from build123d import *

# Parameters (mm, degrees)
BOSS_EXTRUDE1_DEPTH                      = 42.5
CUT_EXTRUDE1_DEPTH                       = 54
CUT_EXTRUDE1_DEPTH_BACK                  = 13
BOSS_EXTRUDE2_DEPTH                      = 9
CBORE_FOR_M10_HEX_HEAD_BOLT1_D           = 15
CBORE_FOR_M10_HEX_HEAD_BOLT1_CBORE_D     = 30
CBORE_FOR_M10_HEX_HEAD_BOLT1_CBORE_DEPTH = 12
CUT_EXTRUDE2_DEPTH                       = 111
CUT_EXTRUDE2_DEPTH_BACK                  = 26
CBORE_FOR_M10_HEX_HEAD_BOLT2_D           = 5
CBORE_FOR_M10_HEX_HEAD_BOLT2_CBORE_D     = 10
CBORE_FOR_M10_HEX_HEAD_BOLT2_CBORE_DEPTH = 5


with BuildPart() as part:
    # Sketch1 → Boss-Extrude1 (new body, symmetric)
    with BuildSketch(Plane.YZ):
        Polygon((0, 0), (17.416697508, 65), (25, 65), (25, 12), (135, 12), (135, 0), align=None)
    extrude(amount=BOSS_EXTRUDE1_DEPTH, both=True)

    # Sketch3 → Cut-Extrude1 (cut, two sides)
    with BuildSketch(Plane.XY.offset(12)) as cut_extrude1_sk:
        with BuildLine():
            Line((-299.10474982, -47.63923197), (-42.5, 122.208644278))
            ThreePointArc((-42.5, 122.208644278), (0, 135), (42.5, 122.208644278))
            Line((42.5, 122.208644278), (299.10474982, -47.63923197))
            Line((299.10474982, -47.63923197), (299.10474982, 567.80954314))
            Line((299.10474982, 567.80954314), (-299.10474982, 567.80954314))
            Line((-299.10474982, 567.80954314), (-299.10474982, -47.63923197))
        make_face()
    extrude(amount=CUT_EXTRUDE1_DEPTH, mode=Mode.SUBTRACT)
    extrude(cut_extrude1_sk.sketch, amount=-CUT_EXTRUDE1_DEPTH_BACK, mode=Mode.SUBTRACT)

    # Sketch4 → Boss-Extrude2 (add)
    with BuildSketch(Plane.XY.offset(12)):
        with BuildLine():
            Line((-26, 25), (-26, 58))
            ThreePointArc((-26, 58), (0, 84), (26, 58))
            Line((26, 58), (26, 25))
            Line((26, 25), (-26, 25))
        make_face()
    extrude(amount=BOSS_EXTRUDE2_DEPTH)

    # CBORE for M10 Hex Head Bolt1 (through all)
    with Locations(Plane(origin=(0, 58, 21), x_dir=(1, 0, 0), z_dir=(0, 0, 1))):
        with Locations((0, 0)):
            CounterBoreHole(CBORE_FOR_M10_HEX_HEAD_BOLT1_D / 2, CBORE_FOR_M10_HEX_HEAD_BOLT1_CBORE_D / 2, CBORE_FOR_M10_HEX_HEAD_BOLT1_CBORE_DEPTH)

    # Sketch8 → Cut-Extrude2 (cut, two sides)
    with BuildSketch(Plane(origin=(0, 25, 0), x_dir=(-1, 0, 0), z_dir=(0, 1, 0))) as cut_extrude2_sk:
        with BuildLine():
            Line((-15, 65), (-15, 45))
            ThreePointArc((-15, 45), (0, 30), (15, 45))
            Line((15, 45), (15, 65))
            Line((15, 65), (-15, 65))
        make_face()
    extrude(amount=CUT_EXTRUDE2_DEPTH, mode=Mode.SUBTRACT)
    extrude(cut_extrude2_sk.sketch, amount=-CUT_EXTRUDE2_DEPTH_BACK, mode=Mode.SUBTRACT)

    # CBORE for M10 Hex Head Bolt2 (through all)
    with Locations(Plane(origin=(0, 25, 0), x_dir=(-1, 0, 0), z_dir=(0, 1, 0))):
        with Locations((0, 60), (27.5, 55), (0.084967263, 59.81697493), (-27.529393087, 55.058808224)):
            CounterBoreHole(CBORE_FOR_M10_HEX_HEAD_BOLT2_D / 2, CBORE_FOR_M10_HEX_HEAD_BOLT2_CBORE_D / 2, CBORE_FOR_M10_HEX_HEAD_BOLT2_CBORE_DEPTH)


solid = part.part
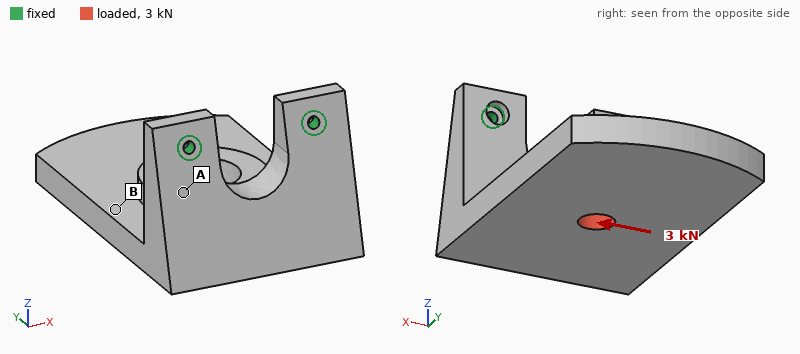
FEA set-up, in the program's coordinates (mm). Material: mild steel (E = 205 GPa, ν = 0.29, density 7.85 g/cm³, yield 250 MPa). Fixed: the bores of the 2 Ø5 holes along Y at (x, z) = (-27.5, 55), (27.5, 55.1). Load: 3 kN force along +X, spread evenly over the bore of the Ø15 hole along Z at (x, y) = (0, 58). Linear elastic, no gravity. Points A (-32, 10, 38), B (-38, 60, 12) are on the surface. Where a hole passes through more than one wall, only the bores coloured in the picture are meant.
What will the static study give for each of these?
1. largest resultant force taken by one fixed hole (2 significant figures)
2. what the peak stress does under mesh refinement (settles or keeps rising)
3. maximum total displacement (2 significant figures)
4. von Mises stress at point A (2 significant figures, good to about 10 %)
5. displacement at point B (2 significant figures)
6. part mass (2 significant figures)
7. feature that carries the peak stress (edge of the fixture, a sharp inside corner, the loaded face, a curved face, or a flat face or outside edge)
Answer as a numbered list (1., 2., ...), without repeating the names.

1. 3.5 kN
2. keeps rising
3. 86 µm
4. 17 MPa
5. 44 µm
6. 1.6 kg
7. edge of the fixture
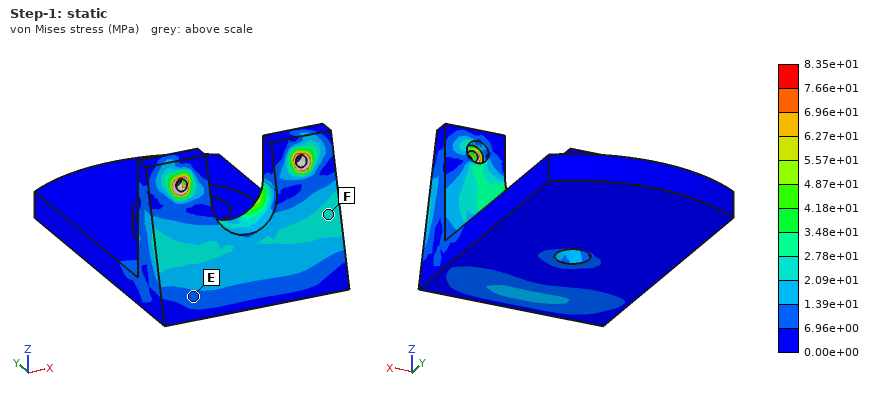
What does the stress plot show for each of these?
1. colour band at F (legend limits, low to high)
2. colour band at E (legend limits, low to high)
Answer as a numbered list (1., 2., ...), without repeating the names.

1. 2.09e+01 to 2.78e+01 MPa
2. 6.96e+00 to 1.39e+01 MPa
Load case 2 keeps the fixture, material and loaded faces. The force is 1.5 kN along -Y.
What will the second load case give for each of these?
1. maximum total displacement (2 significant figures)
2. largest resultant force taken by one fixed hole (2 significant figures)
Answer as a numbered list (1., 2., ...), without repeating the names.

1. 0.28 mm
2. 750 N
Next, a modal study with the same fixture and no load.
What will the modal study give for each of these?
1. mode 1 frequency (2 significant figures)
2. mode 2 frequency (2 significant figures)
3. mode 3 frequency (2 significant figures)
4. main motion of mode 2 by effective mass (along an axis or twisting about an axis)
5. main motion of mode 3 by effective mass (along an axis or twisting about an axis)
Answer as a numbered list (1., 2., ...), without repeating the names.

1. 340 Hz
2. 930 Hz
3. 1700 Hz
4. along X
5. along Y
